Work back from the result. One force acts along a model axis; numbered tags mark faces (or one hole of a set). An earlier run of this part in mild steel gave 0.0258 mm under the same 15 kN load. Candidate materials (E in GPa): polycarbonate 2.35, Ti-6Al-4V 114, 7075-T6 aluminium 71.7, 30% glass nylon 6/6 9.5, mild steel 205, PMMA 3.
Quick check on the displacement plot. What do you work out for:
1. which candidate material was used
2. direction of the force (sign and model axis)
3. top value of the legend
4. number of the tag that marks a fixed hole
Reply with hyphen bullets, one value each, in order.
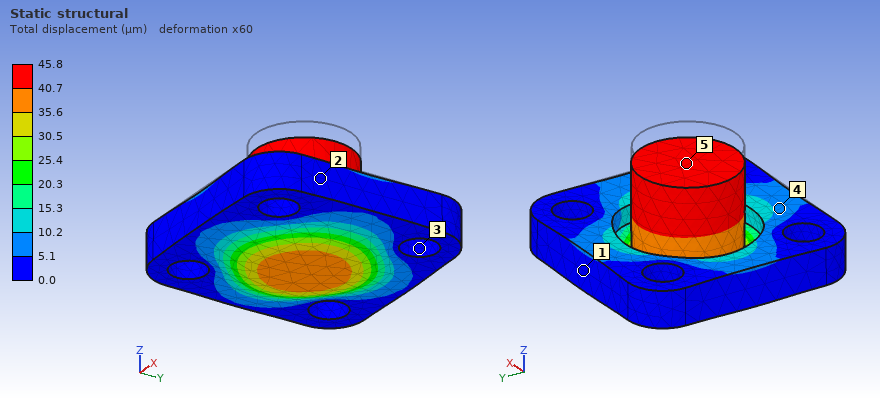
- Ti-6Al-4V
- -Z
- 45.8 µm
- 3
